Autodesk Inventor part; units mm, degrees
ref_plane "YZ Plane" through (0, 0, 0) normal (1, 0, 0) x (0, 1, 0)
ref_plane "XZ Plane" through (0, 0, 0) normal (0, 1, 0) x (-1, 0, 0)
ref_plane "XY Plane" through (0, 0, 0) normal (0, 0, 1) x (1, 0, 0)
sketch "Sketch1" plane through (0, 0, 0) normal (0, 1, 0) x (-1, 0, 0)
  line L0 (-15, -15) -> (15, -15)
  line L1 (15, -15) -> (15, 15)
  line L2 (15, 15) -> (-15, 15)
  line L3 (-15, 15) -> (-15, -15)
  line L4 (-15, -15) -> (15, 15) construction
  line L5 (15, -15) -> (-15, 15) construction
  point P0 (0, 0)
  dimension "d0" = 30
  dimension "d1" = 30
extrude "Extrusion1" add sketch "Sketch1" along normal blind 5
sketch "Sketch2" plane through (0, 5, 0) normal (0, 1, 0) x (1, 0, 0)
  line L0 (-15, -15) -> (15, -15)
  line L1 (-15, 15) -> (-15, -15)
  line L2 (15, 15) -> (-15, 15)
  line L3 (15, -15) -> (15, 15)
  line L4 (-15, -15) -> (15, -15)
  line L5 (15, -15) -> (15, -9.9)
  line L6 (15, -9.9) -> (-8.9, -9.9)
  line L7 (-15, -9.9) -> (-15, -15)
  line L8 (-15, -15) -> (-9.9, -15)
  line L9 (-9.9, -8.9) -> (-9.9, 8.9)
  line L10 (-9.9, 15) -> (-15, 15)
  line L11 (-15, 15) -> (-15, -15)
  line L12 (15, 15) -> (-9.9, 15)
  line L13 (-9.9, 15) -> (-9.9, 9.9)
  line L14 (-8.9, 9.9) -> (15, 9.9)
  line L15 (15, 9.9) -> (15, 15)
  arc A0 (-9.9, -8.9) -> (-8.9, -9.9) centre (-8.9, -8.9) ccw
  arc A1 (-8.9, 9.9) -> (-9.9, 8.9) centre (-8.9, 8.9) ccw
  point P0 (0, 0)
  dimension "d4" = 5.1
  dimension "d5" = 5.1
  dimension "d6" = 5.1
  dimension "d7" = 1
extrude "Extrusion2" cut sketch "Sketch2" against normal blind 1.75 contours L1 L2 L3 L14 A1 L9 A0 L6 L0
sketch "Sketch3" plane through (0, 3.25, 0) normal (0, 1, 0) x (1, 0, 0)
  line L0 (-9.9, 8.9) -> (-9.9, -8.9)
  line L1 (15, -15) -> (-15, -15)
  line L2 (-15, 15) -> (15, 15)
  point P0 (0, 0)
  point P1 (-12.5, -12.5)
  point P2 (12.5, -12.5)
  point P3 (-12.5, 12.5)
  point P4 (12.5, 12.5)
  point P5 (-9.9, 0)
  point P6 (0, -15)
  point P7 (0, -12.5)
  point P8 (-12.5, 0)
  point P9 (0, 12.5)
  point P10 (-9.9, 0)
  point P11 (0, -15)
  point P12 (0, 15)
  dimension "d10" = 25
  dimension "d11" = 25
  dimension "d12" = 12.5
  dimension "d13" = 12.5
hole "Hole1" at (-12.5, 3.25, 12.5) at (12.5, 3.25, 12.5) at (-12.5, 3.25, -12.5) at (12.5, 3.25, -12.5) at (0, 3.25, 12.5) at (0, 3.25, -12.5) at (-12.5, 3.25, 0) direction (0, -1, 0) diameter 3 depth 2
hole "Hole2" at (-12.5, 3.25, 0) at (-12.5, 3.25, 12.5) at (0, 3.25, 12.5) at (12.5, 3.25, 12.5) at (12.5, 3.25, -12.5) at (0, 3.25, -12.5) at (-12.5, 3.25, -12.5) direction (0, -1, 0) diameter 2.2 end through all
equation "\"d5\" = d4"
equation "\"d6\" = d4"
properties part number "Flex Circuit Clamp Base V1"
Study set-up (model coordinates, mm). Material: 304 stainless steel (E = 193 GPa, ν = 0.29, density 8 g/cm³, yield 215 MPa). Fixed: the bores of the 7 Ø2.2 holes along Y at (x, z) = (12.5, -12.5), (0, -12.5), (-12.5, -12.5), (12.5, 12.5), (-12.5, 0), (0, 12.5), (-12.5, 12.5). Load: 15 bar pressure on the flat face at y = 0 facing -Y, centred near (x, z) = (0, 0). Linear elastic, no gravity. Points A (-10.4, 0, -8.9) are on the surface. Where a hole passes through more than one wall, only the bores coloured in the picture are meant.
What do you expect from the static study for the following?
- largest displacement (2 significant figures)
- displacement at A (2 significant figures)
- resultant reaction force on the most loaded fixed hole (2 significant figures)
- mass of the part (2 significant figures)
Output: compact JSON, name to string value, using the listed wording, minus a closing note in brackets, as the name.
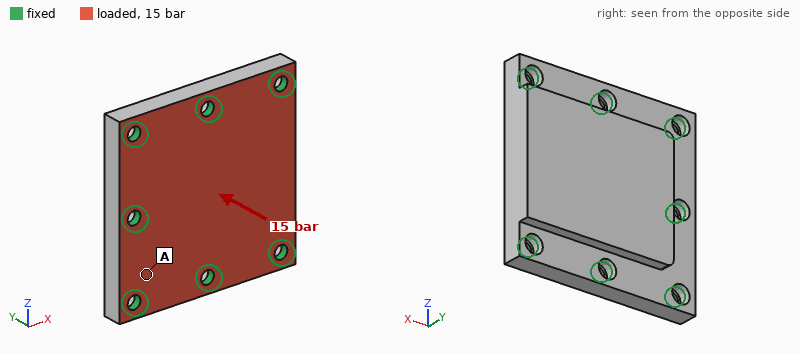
{"largest displacement": "2.5 µm", "displacement at A": "0.59 µm", "resultant reaction force on the most loaded fixed hole": "270 N", "mass of the part": "29 g"}
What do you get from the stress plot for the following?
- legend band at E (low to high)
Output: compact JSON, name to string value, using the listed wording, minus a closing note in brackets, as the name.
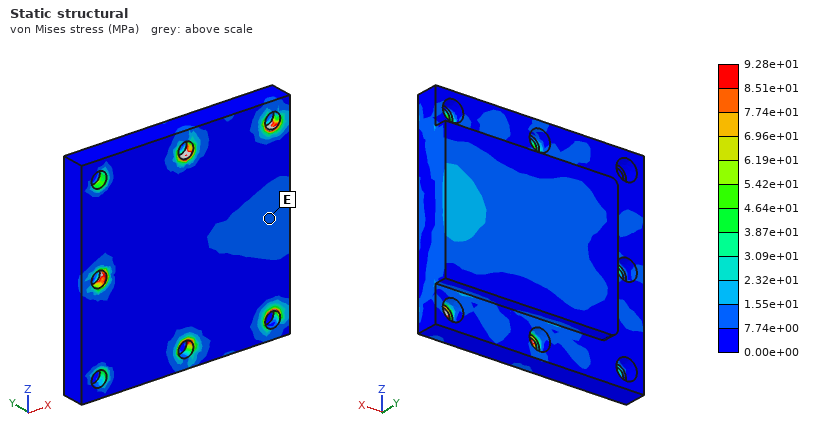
{"legend band at E": "7.74e+00 to 1.55e+01 MPa"}
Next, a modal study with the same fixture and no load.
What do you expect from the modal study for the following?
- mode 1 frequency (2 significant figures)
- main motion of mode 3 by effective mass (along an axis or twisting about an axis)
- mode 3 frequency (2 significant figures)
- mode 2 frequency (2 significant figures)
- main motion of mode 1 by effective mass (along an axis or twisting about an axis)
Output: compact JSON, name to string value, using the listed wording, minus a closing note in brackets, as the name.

{"mode 1 frequency": "24 kHz", "main motion of mode 3 by effective mass": "along Z", "mode 3 frequency": "48 kHz", "mode 2 frequency": "37 kHz", "main motion of mode 1 by effective mass": "along Y"}
